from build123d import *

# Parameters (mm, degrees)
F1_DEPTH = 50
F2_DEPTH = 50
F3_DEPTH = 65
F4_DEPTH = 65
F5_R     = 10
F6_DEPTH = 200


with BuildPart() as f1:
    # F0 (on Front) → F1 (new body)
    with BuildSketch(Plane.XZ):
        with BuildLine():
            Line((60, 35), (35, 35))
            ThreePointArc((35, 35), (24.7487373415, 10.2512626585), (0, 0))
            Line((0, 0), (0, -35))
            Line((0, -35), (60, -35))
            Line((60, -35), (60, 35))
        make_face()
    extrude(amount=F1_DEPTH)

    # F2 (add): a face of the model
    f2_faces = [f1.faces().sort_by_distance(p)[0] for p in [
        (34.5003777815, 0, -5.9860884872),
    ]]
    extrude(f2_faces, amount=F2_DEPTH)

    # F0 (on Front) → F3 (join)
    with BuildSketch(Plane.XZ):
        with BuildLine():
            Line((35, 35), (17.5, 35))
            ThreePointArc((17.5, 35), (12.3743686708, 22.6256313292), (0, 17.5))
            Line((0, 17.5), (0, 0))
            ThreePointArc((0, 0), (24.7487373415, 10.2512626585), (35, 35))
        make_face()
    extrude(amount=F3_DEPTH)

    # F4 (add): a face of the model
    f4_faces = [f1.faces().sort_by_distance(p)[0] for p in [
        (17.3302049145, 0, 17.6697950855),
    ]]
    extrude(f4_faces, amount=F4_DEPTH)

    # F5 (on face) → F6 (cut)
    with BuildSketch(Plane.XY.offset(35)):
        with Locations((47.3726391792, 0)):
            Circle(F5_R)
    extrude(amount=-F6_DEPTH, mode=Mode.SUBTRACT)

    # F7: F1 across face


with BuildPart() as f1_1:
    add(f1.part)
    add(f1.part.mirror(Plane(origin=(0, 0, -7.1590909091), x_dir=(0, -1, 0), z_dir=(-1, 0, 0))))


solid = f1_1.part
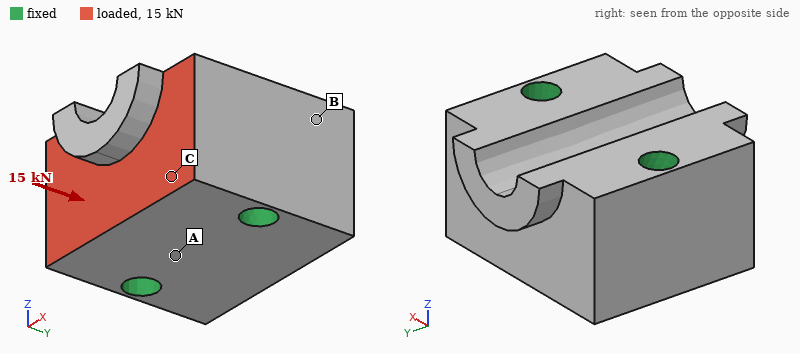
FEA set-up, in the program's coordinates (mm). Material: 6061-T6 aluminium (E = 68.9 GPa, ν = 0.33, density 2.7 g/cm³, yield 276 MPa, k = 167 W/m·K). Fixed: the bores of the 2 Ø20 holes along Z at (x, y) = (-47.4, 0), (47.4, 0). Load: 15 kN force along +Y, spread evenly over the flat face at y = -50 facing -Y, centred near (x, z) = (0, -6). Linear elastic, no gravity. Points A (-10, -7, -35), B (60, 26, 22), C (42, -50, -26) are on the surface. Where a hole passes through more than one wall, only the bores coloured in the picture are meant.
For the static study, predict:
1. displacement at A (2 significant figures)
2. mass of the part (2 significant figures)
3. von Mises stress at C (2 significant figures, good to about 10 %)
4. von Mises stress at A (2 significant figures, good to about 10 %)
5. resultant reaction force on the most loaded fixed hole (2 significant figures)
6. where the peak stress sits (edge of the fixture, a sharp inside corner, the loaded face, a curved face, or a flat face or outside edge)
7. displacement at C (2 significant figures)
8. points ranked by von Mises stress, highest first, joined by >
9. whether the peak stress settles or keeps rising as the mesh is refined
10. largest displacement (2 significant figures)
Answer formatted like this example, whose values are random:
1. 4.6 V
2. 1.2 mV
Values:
1. 1.4 µm
2. 2.1 kg
3. 2.4 MPa
4. 1.2 MPa
5. 7.6 kN
6. edge of the fixture
7. 1.9 µm
8. C > A > B
9. keeps rising
10. 2.7 µm
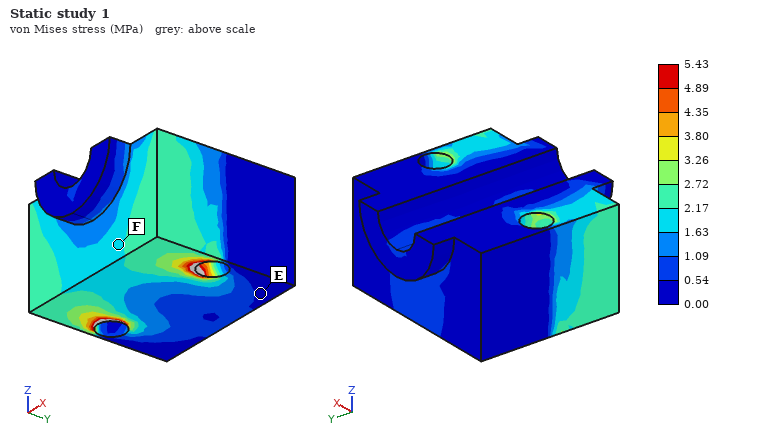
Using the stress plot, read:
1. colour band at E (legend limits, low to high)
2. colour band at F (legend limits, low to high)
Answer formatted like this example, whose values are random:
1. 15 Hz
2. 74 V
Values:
1. 0.00 to 0.54 MPa
2. 1.63 to 2.17 MPa
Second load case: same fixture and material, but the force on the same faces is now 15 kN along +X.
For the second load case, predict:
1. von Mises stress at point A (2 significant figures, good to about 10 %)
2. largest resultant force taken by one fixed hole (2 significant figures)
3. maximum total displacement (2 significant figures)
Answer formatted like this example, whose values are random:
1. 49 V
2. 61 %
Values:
1. 2.6 MPa
2. 10 kN
3. 7.3 µm
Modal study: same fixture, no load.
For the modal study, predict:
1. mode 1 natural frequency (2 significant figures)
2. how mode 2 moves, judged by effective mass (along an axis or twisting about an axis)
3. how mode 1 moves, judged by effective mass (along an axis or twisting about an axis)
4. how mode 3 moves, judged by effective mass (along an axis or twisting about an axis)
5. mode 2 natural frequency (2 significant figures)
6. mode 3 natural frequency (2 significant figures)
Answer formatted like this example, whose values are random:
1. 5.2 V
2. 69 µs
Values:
1. 9700 Hz
2. along Z
3. twisting about X
4. along X
5. 10 kHz
6. 12 kHz
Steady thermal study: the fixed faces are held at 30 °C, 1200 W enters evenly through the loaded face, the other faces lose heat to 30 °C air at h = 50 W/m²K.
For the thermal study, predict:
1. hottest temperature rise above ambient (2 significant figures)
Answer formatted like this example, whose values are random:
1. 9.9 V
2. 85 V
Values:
1. 51 K
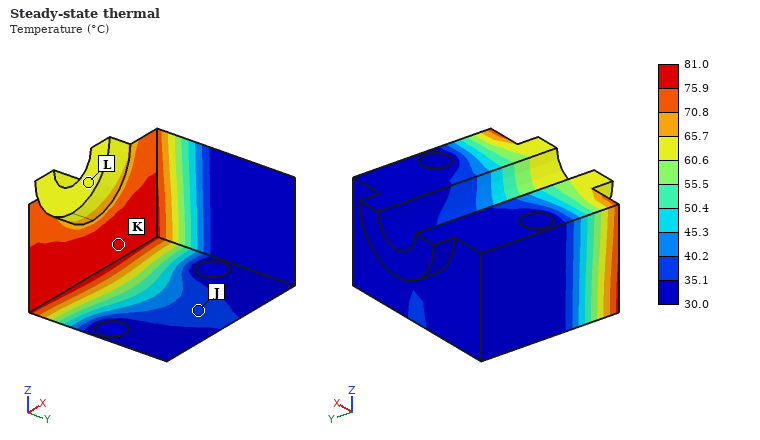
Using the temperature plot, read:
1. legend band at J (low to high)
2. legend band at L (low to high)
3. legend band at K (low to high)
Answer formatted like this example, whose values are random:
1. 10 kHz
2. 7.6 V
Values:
1. 35.1 to 40.2 °C
2. 60.6 to 65.7 °C
3. 75.9 to 81.0 °C
